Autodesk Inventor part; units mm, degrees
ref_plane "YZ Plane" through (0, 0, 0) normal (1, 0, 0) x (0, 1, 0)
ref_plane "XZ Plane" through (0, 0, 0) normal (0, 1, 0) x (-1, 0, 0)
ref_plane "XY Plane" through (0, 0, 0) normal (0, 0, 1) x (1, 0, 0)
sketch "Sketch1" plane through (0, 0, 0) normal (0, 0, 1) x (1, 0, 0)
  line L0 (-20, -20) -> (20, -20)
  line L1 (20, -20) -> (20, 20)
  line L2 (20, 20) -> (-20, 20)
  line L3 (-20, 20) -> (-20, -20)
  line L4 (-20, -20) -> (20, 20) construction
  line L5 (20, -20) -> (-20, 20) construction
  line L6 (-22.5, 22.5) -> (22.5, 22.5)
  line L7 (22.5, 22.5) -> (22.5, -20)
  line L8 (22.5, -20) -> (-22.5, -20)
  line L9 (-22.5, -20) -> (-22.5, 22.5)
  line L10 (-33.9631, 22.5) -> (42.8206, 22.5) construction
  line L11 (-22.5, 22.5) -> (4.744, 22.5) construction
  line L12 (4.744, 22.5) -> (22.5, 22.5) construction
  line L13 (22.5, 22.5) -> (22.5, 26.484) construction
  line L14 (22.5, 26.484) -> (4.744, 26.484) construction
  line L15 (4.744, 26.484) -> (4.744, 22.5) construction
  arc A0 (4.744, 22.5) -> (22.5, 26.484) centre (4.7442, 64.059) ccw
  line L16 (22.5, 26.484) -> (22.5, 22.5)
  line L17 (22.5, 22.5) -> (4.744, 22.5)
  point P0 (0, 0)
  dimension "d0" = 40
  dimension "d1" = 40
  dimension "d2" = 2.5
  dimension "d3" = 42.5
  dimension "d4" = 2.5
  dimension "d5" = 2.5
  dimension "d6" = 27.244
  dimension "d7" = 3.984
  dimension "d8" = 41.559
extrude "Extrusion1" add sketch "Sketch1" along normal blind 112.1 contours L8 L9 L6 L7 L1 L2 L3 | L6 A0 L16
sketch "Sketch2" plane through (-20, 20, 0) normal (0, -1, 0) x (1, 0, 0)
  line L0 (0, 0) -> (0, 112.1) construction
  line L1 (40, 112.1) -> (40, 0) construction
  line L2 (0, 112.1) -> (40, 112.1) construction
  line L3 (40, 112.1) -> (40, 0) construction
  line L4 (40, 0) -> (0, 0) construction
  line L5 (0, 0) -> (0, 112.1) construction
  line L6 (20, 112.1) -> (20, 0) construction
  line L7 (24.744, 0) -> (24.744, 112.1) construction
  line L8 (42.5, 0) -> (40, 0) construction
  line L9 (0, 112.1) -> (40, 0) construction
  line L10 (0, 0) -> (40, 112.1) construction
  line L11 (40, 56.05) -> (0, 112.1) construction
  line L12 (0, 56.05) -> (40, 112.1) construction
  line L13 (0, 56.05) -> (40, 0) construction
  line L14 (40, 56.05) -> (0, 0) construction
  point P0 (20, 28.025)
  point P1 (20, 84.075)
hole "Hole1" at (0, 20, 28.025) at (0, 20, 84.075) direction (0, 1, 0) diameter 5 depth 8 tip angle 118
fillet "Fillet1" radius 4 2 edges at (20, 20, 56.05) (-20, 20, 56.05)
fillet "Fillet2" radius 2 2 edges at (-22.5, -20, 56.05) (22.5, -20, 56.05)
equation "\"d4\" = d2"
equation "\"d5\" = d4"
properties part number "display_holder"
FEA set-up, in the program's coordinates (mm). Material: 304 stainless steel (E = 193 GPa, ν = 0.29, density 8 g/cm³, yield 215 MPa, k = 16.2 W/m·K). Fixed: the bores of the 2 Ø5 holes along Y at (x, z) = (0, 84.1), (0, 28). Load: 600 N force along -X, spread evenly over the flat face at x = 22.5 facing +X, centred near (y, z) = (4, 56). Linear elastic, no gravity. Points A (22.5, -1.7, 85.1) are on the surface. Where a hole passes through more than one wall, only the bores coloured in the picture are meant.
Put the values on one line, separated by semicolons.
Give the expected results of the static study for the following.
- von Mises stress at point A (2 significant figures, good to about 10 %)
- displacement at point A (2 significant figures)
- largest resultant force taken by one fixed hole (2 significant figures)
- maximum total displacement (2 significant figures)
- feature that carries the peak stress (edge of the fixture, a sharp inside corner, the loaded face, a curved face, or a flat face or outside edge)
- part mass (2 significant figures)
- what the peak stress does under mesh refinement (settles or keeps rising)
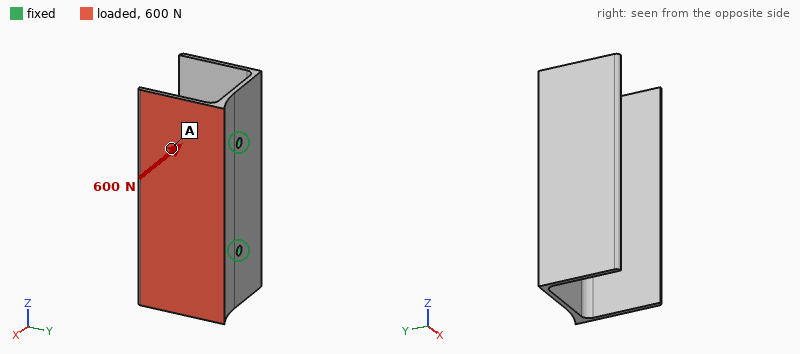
14 MPa; 0.19 mm; 300 N; 0.34 mm; edge of the fixture; 300 g; keeps rising
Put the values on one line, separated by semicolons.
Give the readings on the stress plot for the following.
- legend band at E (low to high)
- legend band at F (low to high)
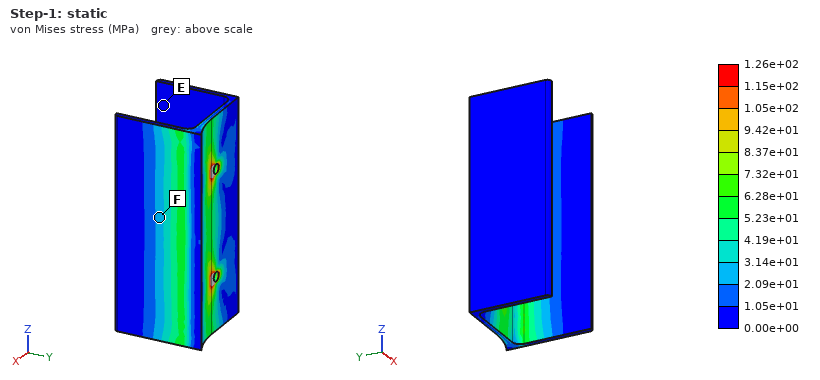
0.00e+00 to 1.05e+01 MPa; 2.09e+01 to 3.14e+01 MPa
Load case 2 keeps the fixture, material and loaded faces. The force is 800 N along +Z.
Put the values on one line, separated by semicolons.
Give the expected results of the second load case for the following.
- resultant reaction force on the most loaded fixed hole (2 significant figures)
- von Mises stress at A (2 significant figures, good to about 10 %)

550 N; 6.8 MPa
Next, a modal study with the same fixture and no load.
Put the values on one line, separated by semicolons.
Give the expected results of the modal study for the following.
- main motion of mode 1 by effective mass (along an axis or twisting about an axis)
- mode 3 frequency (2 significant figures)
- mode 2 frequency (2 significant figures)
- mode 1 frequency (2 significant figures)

along X; 990 Hz; 760 Hz; 610 Hz
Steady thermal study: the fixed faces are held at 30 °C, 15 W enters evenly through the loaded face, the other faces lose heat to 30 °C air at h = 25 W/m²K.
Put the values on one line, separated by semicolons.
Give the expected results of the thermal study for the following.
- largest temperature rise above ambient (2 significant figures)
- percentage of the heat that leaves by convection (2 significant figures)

57 K; 72 %
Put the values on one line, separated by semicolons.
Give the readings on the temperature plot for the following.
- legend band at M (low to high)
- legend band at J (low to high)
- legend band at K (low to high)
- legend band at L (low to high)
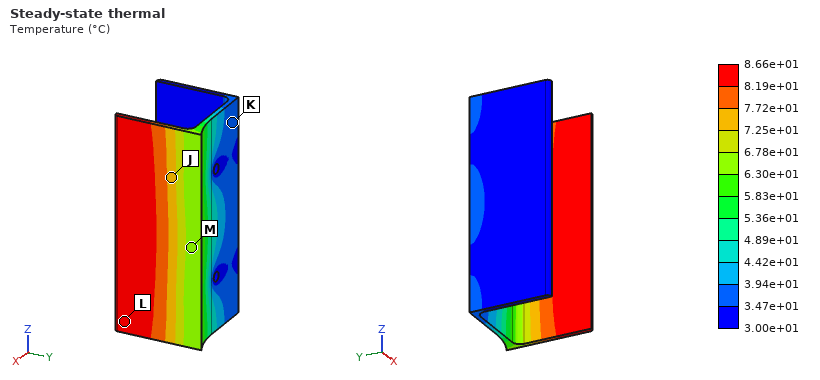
6.30e+01 to 6.78e+01 °C; 7.25e+01 to 7.72e+01 °C; 3.47e+01 to 3.94e+01 °C; 8.19e+01 to 8.66e+01 °C
